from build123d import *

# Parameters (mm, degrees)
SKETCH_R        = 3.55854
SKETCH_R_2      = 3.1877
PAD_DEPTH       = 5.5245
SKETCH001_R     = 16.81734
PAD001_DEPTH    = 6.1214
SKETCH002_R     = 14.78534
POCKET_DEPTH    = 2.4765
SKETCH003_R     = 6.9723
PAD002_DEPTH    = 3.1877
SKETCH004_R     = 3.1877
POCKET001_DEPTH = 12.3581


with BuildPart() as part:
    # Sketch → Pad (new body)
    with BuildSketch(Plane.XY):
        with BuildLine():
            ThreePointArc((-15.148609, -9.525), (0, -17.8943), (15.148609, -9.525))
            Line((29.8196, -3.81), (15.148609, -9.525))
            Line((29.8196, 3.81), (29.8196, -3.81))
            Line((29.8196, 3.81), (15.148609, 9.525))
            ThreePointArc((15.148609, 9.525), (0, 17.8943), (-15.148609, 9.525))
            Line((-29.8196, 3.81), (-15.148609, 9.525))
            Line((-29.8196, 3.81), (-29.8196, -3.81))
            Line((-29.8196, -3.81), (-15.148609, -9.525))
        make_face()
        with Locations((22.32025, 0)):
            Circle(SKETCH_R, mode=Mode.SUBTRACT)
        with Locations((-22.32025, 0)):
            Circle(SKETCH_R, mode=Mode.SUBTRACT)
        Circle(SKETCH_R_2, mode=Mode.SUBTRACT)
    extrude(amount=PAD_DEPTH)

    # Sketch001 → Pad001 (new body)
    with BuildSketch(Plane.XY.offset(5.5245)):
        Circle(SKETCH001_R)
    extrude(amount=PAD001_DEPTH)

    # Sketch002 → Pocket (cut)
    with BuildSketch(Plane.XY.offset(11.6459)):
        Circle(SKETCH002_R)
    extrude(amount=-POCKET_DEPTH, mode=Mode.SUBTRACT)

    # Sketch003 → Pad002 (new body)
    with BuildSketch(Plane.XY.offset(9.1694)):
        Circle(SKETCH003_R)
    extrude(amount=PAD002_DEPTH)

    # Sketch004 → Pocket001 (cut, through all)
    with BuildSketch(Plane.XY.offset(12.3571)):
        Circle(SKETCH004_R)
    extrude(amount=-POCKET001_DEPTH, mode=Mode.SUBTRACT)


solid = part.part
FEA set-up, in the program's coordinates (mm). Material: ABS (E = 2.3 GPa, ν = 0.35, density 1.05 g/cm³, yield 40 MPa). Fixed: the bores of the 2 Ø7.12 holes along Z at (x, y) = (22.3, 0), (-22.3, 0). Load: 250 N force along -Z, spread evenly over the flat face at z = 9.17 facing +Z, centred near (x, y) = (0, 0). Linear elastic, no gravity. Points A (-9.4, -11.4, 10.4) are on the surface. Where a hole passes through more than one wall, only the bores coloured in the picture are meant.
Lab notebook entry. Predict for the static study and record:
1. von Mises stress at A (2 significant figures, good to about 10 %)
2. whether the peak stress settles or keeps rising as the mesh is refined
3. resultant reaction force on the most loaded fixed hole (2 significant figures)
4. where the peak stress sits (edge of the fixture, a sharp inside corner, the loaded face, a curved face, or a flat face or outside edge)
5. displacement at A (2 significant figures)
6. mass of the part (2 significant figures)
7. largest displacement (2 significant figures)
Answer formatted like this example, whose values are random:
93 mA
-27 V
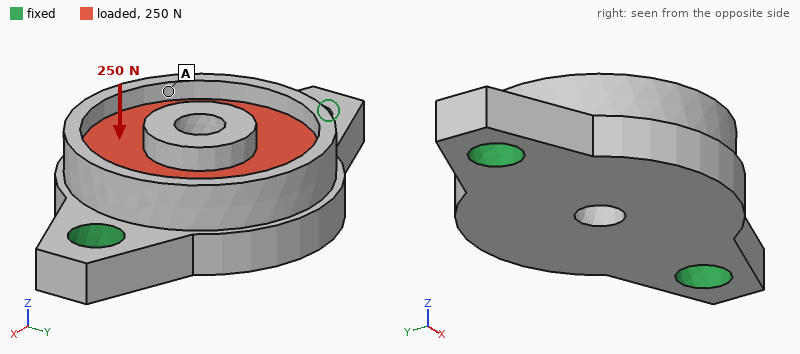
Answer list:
1.2 MPa
keeps rising
150 N
edge of the fixture
41 µm
11 g
57 µm
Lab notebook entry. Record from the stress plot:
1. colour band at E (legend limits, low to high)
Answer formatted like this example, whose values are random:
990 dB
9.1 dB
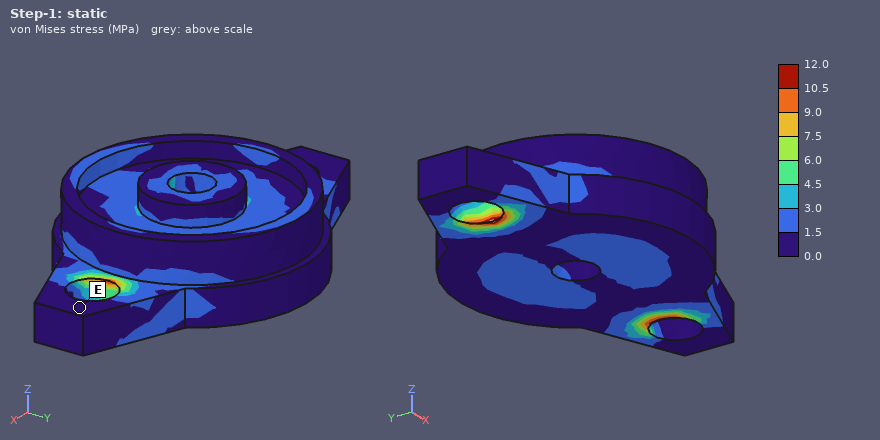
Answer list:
0.0 to 1.5 MPa
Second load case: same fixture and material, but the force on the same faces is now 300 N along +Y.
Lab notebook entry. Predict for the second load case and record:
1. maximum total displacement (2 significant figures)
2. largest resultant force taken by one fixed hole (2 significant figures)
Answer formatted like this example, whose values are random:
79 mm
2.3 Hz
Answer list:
0.15 mm
150 N
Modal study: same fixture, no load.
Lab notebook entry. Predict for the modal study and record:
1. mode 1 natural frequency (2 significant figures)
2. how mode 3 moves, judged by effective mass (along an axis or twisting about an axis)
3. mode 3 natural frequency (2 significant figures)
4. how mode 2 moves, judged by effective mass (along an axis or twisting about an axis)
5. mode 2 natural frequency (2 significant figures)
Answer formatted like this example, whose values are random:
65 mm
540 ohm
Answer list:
2700 Hz
along Y
6600 Hz
along Z
3900 Hz
